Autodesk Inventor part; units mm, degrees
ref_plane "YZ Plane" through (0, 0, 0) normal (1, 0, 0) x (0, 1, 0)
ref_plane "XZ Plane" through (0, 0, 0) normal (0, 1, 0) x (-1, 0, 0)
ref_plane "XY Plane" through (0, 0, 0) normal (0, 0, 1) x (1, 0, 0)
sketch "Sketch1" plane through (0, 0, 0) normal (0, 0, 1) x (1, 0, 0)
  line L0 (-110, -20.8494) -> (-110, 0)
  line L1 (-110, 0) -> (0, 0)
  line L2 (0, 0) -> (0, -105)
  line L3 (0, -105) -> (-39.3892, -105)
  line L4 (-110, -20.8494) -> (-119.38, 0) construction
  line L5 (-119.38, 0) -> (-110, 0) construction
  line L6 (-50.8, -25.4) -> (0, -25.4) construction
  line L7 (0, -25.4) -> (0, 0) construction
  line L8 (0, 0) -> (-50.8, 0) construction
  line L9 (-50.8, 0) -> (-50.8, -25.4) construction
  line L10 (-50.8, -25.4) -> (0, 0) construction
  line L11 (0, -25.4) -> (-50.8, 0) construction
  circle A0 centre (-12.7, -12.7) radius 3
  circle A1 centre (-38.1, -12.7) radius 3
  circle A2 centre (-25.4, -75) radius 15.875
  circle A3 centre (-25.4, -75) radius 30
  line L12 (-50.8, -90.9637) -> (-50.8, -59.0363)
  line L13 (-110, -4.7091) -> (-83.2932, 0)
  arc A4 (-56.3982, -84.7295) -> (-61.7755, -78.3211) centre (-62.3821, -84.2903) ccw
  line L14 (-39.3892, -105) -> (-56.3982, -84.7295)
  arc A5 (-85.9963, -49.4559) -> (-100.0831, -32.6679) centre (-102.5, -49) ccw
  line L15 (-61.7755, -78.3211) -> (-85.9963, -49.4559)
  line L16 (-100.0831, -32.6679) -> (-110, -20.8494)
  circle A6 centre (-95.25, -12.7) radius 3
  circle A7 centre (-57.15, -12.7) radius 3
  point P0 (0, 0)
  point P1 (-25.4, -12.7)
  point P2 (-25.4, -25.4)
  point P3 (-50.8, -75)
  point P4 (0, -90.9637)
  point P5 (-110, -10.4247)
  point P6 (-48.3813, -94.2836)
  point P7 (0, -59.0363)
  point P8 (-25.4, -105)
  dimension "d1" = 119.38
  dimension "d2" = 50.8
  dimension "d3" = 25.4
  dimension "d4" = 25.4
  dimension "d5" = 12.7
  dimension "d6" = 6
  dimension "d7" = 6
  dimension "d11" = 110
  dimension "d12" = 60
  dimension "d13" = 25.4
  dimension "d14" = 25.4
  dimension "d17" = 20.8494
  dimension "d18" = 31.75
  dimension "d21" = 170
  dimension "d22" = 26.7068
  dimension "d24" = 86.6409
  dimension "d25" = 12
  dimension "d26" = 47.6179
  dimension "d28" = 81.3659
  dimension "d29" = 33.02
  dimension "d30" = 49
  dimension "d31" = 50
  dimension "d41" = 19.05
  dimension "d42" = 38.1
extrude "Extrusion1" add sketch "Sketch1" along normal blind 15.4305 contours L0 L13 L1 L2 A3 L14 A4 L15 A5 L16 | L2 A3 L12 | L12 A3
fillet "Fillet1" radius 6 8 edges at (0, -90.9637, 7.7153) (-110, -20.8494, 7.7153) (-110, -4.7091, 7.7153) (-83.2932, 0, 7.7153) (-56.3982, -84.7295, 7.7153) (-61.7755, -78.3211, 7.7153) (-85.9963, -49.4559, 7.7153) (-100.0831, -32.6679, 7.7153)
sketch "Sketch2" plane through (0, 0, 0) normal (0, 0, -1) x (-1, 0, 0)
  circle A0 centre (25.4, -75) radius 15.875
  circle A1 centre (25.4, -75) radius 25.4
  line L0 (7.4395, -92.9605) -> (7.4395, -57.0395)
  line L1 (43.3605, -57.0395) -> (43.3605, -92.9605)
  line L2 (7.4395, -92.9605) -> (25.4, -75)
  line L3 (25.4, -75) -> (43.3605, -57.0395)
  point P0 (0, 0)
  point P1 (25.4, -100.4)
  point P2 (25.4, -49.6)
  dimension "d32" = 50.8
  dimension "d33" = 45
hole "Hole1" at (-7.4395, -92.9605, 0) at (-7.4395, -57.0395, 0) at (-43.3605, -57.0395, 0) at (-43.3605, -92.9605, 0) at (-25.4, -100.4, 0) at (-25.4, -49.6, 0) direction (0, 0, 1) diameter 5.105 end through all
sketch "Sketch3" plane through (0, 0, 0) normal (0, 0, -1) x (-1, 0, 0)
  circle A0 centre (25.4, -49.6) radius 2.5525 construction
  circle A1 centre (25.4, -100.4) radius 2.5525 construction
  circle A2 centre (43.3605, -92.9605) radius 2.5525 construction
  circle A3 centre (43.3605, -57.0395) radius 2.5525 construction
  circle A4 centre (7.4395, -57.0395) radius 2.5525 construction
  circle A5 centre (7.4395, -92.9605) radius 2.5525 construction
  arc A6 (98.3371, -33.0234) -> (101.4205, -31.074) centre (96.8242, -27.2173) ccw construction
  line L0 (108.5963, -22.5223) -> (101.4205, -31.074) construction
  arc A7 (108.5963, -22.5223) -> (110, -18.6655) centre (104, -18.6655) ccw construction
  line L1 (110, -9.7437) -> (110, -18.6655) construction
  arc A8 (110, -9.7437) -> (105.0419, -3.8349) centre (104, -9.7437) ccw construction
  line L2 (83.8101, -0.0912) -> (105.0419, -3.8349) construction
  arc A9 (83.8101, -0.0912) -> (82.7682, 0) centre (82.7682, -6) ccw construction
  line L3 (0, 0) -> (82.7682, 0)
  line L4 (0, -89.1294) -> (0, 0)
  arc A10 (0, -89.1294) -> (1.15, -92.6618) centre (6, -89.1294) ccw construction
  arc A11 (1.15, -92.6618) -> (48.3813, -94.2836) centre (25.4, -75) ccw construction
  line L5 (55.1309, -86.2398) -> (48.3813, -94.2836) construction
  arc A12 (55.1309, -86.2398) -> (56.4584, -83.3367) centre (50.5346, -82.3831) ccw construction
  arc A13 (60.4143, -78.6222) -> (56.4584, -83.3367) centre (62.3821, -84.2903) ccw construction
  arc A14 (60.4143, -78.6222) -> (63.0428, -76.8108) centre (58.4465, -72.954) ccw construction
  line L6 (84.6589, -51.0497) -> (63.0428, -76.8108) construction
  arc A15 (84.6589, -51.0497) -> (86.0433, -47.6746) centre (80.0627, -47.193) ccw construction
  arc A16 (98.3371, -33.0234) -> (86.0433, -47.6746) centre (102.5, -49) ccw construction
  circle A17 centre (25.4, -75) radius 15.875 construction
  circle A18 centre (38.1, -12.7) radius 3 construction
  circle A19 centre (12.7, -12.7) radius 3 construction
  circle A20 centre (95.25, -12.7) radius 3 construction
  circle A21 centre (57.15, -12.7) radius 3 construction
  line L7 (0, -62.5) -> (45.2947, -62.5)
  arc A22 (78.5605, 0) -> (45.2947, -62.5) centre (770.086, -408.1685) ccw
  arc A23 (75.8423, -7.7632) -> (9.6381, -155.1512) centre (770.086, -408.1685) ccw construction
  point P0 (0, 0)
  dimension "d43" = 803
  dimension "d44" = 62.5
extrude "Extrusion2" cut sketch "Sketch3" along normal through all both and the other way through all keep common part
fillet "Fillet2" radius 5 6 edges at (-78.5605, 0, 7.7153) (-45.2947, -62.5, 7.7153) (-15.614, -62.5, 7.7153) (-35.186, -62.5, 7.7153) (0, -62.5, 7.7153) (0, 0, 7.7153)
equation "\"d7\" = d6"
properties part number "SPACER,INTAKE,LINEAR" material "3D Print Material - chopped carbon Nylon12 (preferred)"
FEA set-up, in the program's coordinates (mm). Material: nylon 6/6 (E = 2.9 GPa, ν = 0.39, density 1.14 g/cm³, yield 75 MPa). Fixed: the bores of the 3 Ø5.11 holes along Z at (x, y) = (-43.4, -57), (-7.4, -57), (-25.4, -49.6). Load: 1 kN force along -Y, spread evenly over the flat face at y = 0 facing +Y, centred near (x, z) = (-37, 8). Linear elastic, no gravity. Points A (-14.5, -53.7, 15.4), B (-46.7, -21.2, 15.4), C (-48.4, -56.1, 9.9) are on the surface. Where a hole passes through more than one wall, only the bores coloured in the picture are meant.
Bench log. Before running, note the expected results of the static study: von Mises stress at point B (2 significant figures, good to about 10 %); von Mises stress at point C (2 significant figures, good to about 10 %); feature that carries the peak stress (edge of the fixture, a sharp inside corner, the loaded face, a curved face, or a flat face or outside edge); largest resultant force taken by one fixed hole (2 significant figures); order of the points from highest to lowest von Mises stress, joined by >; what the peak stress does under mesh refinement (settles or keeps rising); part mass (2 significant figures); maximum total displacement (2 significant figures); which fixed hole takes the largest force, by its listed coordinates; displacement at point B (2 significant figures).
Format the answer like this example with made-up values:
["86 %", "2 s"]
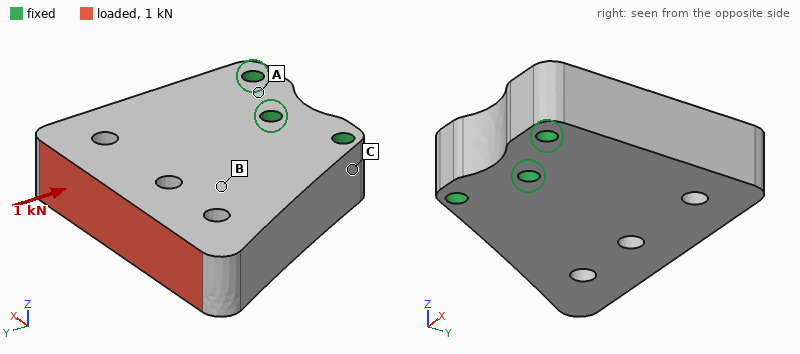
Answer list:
["1.7 MPa", "3.0 MPa", "edge of the fixture", "620 N", "C > B > A", "keeps rising", "64 g", "73 µm", "(-43.4, -57)", "35 µm"]
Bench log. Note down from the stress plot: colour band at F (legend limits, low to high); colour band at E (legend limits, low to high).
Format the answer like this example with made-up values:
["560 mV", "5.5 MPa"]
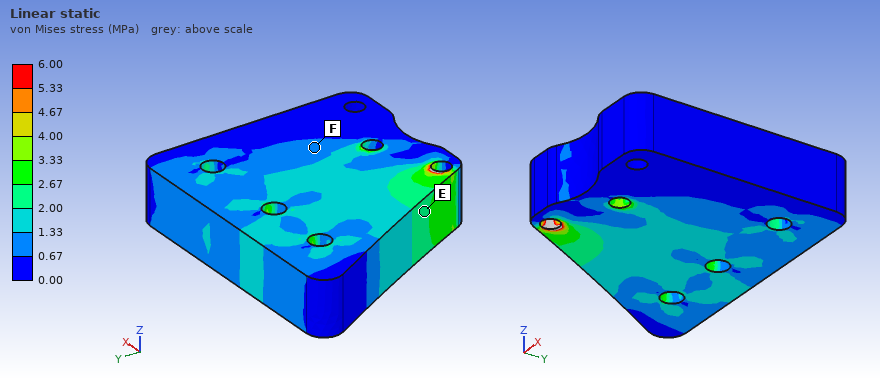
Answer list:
["0.67 to 1.33 MPa", "2.00 to 2.67 MPa"]
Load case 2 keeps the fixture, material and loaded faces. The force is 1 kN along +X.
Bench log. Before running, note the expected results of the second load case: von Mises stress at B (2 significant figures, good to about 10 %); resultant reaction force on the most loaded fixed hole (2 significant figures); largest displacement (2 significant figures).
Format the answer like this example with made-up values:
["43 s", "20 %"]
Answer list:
["2.0 MPa", "1.3 kN", "0.27 mm"]
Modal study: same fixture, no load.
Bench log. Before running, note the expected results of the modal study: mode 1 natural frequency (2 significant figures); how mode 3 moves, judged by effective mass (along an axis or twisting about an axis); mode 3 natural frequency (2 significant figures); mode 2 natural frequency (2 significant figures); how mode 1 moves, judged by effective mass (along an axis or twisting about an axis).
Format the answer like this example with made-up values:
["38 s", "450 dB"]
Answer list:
["1100 Hz", "along X", "2300 Hz", "1900 Hz", "along Z"]
